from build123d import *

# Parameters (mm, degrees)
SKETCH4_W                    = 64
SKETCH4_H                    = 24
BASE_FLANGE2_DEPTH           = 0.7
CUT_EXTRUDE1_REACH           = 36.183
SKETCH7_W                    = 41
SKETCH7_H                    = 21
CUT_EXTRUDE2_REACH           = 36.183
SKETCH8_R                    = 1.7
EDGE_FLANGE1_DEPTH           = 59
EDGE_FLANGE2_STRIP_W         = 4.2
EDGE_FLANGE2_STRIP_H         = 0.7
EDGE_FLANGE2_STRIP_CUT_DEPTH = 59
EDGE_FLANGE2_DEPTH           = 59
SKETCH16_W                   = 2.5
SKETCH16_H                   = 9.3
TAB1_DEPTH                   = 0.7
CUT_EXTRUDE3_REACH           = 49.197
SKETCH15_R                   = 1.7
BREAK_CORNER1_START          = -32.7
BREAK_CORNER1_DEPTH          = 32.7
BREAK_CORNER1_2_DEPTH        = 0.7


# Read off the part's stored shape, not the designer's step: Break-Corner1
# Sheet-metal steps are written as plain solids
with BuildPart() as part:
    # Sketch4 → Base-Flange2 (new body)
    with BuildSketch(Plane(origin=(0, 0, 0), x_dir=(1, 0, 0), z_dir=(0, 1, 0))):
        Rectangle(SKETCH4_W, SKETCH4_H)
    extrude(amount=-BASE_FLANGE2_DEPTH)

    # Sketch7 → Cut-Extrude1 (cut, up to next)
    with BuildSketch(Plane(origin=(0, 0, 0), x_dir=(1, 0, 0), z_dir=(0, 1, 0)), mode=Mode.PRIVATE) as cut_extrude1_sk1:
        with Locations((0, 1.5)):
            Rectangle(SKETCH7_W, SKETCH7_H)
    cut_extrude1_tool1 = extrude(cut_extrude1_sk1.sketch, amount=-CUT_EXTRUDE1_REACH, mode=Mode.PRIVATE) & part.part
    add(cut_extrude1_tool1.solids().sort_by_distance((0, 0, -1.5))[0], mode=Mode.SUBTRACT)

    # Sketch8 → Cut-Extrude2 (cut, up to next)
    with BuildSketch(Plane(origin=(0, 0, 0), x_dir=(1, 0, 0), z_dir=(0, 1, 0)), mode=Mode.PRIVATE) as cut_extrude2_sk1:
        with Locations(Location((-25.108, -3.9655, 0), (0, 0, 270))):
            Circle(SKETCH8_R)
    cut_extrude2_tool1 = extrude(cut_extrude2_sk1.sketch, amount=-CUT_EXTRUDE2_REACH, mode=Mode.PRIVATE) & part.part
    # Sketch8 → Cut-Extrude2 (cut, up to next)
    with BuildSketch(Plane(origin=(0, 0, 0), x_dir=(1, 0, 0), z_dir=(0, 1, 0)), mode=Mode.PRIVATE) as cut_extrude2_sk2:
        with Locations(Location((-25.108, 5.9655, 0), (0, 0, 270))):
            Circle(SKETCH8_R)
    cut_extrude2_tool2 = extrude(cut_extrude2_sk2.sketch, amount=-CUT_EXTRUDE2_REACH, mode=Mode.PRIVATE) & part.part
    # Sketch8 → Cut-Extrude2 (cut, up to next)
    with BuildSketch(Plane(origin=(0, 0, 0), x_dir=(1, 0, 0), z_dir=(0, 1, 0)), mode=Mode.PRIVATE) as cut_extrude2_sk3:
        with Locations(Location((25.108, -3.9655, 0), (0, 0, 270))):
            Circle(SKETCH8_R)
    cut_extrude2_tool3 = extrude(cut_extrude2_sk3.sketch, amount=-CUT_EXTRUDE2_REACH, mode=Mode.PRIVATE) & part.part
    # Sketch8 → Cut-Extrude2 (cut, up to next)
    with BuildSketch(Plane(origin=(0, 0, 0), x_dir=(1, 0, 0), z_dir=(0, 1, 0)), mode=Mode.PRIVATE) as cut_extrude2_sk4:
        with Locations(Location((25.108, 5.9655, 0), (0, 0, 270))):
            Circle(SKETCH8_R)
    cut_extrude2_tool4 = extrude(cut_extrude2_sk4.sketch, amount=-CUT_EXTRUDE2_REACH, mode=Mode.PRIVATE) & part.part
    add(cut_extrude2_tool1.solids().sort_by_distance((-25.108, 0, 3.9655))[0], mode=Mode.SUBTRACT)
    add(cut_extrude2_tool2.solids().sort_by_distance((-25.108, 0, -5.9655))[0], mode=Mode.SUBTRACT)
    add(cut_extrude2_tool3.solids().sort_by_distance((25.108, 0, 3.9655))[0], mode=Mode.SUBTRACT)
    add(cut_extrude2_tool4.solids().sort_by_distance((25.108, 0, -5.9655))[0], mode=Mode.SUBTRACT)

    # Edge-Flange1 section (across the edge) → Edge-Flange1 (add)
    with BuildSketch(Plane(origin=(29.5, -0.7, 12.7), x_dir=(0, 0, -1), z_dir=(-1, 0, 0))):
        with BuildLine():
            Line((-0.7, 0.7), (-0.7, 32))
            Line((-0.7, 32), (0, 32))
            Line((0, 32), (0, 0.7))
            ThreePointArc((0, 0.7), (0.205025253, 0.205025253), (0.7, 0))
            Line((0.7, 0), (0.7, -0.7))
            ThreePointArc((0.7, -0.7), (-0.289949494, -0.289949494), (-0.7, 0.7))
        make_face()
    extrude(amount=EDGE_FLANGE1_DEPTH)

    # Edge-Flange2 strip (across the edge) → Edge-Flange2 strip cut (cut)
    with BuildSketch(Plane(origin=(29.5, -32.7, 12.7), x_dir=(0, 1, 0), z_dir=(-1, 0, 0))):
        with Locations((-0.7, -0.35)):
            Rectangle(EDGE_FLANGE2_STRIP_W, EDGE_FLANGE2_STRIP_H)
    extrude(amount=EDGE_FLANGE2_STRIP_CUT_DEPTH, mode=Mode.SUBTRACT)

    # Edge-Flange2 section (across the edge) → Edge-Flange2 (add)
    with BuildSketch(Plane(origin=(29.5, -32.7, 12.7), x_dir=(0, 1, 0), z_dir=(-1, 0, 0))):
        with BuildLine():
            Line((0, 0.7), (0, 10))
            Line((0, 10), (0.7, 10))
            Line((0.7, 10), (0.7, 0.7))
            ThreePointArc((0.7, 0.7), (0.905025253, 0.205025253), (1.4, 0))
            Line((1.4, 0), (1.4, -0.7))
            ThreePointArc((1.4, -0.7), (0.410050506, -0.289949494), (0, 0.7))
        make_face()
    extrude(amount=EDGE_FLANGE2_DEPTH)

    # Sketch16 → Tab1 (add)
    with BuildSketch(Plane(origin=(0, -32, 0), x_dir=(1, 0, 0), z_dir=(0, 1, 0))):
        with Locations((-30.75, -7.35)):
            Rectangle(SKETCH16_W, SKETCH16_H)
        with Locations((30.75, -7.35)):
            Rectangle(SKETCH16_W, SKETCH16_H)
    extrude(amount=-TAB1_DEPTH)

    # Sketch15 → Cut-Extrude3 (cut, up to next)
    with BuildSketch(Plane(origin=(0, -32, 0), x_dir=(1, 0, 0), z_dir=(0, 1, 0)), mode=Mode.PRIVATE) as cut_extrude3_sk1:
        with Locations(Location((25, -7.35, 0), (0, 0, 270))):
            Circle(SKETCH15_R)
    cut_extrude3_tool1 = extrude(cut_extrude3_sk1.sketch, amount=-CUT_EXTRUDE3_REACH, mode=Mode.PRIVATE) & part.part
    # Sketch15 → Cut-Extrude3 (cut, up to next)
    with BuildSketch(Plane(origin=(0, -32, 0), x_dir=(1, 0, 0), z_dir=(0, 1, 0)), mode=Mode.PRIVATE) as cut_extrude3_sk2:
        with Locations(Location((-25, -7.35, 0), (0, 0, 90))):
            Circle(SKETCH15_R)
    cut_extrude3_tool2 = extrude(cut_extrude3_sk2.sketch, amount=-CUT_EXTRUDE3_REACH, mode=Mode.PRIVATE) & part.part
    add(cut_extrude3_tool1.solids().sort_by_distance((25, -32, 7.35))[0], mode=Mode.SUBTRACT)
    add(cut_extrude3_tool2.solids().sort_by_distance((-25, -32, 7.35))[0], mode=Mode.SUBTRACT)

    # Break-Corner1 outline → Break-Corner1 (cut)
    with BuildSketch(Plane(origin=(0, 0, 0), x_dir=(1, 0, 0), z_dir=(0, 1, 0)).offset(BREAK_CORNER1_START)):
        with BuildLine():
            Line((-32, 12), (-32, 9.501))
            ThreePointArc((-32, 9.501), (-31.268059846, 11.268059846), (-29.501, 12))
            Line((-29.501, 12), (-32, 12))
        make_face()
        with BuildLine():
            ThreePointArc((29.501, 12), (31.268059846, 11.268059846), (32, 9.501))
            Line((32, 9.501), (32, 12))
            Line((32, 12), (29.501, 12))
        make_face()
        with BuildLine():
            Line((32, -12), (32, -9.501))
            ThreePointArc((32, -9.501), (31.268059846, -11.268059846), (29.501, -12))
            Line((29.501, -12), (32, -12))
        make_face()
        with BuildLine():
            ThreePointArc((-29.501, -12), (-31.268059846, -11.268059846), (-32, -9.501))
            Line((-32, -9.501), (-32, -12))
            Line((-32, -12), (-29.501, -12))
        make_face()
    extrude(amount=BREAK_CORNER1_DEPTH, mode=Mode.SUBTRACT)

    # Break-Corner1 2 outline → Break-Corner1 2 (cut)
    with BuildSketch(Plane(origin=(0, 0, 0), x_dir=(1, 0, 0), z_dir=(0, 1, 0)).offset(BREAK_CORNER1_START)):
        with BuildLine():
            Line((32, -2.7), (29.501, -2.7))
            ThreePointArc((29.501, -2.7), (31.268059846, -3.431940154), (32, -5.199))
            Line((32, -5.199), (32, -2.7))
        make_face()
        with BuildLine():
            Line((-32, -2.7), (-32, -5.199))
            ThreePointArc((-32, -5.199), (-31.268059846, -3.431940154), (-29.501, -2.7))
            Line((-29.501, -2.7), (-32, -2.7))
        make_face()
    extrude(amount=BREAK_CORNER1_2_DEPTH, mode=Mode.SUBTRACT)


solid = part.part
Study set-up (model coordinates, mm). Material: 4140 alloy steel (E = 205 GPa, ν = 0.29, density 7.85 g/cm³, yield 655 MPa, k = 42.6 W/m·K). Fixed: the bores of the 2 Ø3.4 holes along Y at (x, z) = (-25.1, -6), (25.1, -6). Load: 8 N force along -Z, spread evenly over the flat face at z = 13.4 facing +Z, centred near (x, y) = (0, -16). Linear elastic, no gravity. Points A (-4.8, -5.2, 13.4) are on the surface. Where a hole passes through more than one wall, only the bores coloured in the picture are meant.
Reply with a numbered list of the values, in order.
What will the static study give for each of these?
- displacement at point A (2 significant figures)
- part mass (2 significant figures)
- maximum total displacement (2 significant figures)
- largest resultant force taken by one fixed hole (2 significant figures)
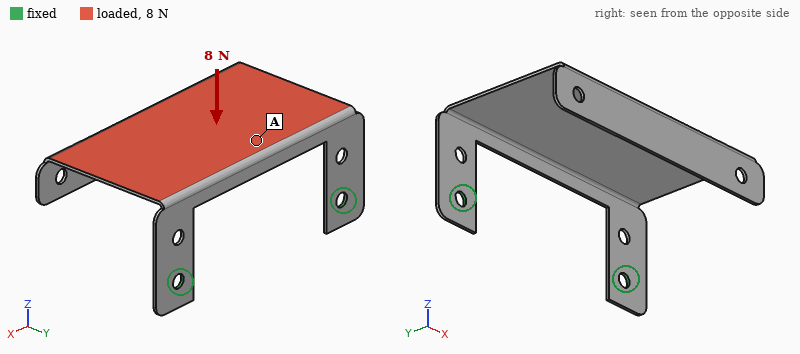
1. 0.20 mm
2. 17 g
3. 0.74 mm
4. 4.2 N
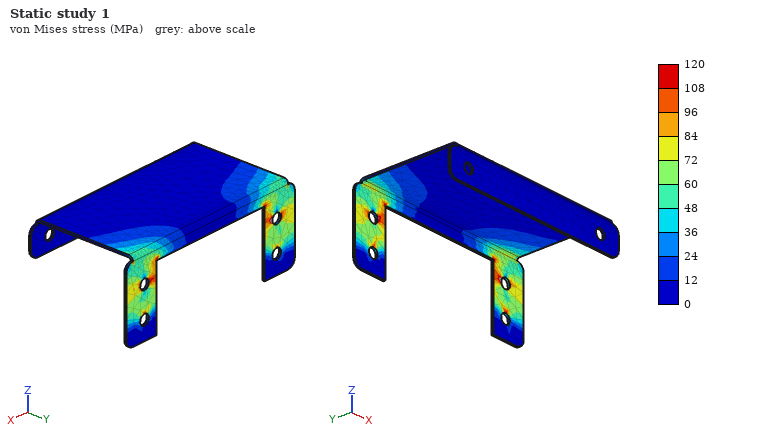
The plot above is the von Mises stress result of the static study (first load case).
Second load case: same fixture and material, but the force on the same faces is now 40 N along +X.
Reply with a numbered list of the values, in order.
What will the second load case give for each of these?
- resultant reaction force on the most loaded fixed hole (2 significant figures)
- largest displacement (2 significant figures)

1. 23 N
2. 0.35 mm
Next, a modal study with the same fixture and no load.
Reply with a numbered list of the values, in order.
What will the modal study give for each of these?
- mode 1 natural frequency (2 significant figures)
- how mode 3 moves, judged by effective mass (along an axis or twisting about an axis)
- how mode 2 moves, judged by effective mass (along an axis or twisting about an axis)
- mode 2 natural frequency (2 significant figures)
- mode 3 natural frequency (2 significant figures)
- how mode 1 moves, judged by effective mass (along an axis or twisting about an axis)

1. 140 Hz
2. along Y
3. along X
4. 400 Hz
5. 540 Hz
6. along Z
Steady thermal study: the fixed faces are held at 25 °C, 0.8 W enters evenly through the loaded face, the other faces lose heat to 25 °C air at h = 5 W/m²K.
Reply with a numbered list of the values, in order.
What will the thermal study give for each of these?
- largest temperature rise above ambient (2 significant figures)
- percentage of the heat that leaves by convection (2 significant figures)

1. 20 K
2. 46 %
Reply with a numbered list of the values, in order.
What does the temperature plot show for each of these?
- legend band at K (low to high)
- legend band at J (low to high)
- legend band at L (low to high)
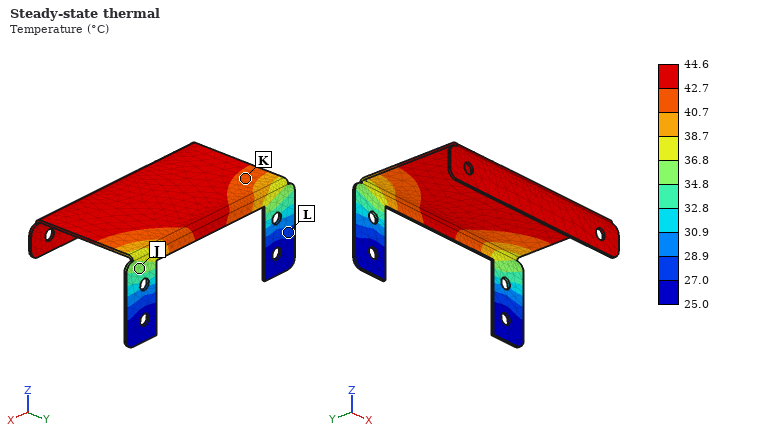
1. 40.7 to 42.7 °C
2. 34.8 to 36.8 °C
3. 27.0 to 28.9 °C
